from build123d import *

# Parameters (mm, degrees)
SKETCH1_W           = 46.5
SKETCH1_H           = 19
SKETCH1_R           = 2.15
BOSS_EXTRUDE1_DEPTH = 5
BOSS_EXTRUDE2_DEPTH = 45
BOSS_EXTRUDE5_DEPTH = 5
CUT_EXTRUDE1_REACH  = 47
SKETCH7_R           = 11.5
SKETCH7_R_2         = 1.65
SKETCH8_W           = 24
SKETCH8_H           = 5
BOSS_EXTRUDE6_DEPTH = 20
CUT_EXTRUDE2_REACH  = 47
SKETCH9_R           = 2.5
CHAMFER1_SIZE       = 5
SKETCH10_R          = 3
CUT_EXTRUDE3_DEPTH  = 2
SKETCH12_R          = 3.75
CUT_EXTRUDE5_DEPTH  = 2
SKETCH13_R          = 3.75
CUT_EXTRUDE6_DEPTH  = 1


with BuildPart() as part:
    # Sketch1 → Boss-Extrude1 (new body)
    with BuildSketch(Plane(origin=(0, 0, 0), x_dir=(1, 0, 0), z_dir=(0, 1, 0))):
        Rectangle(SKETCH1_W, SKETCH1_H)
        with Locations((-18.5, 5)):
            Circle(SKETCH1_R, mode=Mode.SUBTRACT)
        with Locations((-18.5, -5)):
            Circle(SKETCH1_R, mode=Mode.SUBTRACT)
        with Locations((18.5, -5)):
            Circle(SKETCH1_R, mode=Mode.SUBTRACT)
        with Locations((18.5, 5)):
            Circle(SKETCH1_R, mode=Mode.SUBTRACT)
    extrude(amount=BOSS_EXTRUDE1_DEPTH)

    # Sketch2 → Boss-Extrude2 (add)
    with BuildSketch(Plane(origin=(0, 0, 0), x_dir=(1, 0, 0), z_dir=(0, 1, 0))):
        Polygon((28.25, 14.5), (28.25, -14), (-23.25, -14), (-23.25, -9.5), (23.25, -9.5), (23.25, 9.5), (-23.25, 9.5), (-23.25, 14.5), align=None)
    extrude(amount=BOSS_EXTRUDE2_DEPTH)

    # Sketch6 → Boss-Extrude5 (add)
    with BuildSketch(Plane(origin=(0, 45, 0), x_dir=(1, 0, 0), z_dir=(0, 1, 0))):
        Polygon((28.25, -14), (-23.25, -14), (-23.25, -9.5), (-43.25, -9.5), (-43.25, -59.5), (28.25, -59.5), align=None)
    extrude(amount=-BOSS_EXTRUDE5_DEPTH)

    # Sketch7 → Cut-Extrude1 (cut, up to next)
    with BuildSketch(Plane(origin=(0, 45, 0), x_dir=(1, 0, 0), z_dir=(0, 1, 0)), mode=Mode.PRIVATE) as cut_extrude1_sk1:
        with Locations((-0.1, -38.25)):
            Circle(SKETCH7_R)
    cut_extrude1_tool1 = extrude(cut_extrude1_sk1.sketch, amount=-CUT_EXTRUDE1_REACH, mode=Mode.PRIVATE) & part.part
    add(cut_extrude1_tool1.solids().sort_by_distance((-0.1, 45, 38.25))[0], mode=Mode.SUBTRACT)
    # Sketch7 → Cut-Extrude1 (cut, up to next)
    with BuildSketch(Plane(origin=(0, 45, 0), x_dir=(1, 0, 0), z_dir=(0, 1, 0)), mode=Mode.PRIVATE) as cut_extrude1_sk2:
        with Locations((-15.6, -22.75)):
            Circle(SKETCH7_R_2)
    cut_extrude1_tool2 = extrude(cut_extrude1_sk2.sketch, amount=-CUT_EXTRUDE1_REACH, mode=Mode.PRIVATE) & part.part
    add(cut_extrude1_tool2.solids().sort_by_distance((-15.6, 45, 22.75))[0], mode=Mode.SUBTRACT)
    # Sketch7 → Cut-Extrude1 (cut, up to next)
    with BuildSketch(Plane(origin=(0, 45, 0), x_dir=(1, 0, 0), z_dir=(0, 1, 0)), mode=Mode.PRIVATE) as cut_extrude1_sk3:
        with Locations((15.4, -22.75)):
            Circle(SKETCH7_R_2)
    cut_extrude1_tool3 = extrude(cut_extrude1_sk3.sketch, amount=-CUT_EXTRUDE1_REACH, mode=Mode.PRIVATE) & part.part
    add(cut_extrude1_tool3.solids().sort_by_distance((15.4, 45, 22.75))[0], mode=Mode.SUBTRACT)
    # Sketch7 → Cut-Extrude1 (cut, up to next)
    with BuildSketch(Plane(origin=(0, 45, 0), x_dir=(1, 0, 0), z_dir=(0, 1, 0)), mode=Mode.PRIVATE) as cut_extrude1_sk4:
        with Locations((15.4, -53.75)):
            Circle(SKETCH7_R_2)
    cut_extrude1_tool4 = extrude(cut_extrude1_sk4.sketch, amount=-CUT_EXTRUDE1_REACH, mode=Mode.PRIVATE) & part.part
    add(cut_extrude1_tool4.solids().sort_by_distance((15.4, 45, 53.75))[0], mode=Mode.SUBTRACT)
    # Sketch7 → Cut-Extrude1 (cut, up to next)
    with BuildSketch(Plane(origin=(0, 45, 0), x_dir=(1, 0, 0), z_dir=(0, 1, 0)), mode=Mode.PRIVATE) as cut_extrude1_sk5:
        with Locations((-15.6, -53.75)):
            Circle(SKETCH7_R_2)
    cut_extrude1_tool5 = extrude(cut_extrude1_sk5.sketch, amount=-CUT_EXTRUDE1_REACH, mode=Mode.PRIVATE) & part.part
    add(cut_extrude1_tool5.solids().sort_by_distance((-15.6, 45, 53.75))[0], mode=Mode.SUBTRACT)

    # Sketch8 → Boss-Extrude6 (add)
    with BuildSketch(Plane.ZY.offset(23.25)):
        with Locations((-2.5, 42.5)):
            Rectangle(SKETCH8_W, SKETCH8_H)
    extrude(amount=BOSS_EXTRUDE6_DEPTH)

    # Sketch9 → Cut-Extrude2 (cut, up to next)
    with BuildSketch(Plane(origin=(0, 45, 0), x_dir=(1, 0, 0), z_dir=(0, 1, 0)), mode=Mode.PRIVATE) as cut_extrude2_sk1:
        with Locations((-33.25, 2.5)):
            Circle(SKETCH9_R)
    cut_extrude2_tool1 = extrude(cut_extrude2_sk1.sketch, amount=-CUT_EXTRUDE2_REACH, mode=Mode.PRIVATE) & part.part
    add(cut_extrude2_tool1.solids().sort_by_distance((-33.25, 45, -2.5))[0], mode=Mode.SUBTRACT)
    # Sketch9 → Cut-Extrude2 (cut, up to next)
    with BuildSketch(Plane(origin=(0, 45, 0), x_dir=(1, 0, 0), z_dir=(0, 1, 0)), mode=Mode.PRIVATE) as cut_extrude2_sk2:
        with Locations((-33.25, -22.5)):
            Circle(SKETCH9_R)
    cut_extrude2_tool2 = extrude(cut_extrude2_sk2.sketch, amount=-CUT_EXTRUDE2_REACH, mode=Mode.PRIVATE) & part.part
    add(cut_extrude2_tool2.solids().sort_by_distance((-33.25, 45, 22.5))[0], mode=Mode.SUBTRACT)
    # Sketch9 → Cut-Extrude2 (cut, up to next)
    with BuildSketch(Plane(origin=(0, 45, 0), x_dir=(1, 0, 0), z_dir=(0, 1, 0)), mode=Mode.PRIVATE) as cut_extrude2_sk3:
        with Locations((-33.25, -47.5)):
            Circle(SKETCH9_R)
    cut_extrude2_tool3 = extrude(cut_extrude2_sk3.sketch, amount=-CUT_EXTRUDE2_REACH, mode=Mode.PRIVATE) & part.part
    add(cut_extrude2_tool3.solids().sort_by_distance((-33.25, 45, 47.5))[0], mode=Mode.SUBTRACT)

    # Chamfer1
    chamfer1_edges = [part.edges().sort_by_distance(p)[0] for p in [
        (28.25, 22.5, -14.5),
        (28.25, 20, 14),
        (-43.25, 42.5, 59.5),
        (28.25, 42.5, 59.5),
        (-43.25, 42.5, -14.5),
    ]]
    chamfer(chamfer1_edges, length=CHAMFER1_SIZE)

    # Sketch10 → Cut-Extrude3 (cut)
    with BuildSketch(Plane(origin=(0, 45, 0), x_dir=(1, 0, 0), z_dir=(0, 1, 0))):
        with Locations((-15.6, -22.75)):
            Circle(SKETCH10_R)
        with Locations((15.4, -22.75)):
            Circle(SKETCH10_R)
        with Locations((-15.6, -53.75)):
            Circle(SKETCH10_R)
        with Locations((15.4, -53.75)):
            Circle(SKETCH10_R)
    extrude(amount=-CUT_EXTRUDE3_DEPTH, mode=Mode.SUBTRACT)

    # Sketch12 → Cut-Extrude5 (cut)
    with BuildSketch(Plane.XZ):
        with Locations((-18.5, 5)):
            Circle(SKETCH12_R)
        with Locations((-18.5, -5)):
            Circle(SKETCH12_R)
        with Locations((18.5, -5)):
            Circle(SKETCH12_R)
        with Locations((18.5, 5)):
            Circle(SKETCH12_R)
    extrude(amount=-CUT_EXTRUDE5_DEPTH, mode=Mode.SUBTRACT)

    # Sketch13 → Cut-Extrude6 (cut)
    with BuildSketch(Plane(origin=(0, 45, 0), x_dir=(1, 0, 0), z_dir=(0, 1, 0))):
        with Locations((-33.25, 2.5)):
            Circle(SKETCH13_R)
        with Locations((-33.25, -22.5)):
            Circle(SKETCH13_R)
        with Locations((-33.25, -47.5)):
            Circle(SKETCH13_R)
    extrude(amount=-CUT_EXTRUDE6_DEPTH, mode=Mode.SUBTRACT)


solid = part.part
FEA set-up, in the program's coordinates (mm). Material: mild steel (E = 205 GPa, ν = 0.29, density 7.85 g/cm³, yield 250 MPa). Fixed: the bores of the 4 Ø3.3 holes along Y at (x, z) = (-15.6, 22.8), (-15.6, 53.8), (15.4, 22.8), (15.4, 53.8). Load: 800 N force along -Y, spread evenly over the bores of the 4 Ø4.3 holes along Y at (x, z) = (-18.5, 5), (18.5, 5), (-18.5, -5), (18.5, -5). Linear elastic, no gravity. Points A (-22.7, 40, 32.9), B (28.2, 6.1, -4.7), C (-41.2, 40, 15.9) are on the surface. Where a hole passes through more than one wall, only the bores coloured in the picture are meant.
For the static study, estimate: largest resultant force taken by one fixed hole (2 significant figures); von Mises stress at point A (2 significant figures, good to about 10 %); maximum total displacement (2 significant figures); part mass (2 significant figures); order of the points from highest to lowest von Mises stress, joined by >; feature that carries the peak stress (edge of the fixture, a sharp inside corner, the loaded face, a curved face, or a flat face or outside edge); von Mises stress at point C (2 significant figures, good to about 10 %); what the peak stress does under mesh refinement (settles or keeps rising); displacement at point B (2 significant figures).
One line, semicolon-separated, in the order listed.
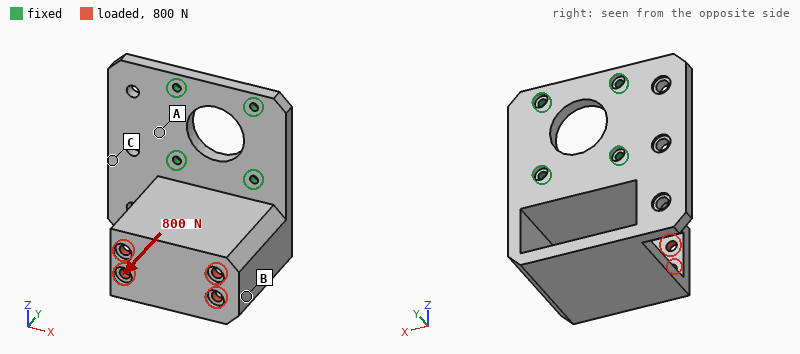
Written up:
700 N; 18 MPa; 0.13 mm; 360 g; C > A > B; edge of the fixture; 34 MPa; keeps rising; 0.10 mm
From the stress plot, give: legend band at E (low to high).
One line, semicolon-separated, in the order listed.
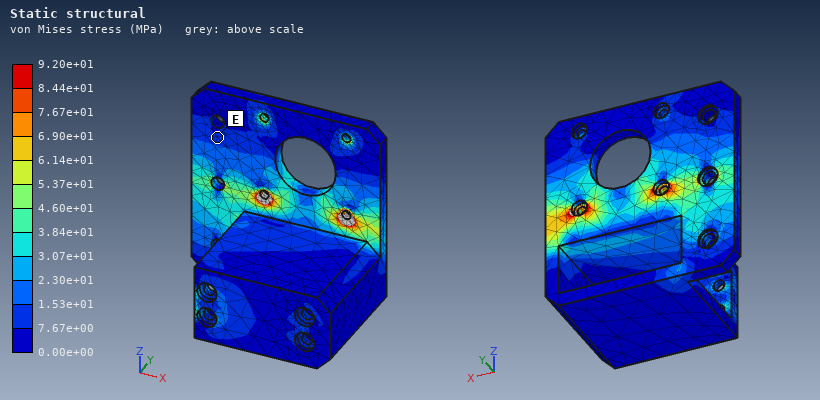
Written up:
7.67e+00 to 1.53e+01 MPa
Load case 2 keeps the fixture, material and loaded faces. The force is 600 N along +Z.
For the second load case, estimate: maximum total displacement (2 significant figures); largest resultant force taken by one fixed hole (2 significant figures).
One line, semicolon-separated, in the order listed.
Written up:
0.21 mm; 740 N
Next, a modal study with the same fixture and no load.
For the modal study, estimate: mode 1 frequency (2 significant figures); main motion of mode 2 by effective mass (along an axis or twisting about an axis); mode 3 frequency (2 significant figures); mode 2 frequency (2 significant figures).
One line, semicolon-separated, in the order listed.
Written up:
750 Hz; along X; 3600 Hz; 2300 Hz
